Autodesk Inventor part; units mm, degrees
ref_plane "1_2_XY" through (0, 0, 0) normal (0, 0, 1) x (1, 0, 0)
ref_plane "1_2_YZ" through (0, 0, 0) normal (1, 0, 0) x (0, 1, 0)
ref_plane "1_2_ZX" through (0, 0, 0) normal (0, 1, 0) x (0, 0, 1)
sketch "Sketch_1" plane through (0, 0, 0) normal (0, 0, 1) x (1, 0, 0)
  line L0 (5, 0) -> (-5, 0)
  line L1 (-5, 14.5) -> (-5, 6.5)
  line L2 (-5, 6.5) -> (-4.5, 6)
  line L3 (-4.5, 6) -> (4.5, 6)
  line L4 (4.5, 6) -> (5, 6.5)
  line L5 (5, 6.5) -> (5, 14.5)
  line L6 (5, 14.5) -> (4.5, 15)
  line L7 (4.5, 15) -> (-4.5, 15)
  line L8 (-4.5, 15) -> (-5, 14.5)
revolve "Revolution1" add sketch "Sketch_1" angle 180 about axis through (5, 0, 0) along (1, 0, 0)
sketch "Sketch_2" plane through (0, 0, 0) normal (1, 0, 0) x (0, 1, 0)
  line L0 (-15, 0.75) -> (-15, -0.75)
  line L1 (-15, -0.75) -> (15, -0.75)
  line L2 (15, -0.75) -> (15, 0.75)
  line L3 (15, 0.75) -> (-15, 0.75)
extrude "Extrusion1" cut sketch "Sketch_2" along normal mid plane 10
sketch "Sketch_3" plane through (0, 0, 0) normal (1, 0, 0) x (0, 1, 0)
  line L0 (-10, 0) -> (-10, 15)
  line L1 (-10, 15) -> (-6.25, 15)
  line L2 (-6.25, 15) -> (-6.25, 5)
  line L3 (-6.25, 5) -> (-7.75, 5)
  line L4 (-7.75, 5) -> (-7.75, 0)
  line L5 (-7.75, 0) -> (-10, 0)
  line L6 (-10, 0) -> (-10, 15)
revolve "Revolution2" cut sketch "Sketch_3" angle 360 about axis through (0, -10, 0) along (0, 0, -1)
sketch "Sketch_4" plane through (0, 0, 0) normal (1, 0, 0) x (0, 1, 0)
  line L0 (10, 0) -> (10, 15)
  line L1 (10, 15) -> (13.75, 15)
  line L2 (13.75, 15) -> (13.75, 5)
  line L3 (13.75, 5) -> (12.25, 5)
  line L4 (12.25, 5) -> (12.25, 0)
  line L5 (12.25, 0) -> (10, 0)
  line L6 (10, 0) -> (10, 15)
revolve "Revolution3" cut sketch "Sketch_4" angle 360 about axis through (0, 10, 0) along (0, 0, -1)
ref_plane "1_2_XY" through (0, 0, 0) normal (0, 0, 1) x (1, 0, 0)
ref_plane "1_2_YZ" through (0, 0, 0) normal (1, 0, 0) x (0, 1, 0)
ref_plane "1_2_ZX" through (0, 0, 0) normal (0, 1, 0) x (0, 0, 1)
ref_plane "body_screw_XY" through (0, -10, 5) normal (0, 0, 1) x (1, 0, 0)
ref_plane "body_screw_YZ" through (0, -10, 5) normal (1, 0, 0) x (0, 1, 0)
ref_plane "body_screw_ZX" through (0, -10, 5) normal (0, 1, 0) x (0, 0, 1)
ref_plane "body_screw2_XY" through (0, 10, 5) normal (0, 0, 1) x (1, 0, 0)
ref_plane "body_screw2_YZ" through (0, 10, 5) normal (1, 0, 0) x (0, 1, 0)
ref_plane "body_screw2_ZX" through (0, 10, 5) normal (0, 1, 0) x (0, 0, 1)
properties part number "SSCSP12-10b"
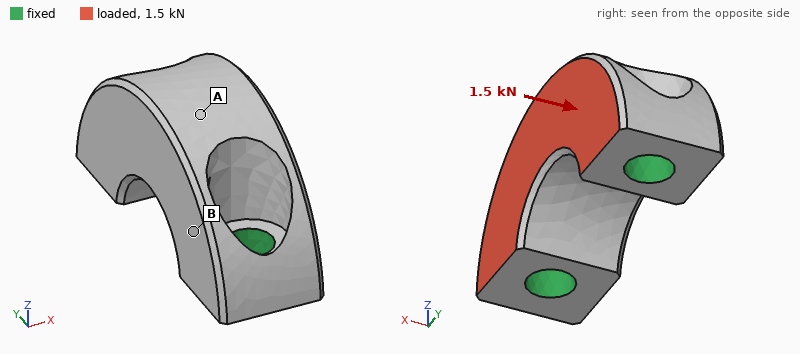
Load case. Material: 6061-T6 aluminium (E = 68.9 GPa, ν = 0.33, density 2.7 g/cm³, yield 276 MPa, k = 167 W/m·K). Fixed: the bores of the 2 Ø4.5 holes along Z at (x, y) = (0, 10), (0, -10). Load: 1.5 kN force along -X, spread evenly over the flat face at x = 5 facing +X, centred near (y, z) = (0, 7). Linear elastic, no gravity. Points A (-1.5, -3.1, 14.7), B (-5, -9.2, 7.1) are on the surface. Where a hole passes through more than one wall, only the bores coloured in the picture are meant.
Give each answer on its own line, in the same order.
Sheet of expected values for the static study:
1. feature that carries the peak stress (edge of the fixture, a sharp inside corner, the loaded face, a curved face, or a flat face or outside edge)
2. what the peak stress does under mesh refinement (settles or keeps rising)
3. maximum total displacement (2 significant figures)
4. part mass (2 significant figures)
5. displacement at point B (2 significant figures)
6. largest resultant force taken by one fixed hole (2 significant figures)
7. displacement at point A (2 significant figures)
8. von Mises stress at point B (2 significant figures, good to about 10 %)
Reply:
edge of the fixture
keeps rising
19 µm
5.8 g
6.5 µm
750 N
17 µm
24 MPa
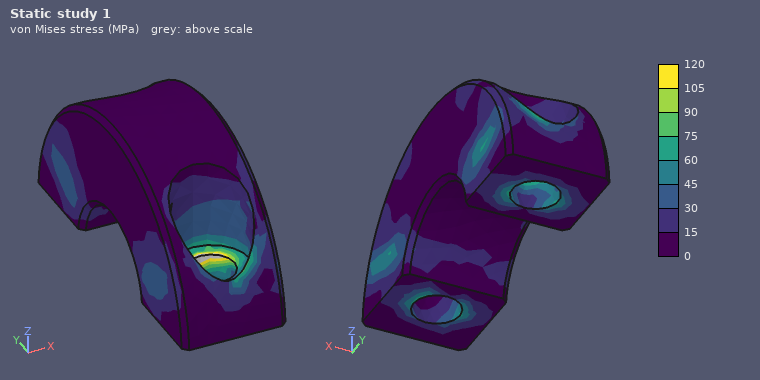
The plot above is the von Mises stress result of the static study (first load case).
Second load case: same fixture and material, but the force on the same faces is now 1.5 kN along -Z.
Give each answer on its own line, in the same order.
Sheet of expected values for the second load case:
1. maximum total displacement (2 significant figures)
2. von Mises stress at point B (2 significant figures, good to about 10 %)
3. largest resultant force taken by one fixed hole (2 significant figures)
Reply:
16 µm
17 MPa
780 N
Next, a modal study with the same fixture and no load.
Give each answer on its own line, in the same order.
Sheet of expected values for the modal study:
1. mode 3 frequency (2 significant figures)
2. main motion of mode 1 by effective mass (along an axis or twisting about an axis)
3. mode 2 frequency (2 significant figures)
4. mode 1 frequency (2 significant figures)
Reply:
50 kHz
along X
49 kHz
22 kHz
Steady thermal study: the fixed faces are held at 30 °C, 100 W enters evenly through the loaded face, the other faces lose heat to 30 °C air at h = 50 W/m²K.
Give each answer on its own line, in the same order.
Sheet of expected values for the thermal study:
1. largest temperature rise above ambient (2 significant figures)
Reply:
39 K
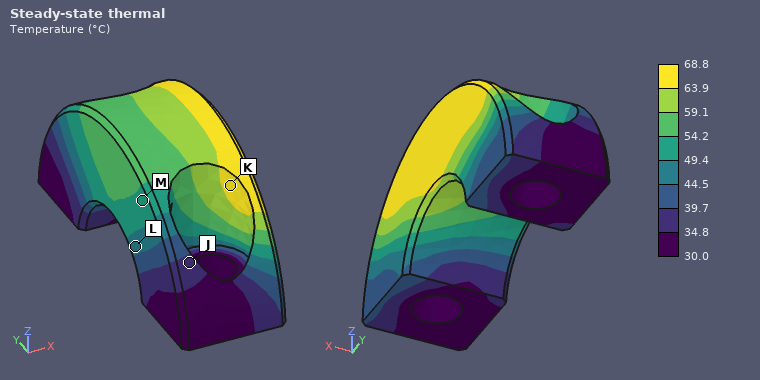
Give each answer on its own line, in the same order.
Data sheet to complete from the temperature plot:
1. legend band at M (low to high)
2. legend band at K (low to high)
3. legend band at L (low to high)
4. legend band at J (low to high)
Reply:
49.4 to 54.2 °C
63.9 to 68.8 °C
44.5 to 49.4 °C
34.8 to 39.7 °C
